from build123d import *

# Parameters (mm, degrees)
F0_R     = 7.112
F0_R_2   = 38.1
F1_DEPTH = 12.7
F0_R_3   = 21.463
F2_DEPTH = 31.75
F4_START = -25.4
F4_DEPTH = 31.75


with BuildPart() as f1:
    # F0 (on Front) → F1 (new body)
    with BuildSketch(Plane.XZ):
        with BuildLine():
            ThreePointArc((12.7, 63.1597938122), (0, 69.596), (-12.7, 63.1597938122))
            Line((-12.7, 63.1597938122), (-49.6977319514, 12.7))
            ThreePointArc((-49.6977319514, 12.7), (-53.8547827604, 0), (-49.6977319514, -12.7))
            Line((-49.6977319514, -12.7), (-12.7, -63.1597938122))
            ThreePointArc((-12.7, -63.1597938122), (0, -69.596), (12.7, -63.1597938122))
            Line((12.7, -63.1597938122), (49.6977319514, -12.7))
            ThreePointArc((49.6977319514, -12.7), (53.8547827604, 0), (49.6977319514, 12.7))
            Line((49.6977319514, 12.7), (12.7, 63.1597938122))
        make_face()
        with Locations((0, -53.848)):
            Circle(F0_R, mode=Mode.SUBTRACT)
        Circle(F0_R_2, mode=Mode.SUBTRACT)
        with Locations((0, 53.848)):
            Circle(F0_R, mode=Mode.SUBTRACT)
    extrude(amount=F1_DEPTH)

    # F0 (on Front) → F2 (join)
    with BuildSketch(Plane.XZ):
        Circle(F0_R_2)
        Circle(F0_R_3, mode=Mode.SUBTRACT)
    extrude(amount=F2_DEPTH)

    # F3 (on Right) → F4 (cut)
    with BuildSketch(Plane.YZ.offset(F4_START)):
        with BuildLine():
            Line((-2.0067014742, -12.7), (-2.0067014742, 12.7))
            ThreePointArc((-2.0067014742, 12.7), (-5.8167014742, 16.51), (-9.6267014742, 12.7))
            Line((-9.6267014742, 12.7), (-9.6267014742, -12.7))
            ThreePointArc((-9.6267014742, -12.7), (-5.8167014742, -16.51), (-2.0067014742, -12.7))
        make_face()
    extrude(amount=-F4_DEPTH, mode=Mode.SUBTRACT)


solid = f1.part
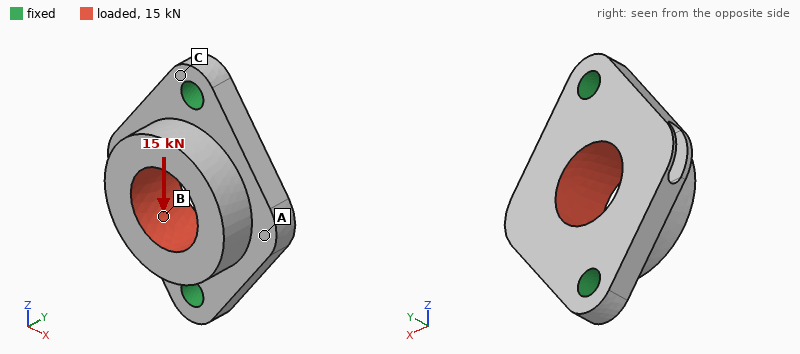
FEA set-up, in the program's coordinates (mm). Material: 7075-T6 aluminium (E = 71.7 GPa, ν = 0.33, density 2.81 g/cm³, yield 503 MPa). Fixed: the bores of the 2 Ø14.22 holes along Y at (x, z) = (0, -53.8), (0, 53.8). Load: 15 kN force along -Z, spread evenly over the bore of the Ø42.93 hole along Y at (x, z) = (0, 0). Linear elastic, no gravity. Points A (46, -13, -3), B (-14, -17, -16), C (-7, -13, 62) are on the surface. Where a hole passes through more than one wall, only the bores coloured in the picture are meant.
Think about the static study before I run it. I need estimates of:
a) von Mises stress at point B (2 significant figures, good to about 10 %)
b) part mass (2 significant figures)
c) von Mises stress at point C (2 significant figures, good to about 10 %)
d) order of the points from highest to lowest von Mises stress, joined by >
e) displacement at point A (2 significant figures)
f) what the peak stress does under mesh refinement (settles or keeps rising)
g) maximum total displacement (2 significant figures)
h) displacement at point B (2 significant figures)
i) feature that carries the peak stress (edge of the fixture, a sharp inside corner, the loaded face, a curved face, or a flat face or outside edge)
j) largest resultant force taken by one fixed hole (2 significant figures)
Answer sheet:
9.4 MPa
410 g
5.5 MPa
B > C > A
6.1 µm
keeps rising
11 µm
8.3 µm
edge of the fixture
7.7 kN
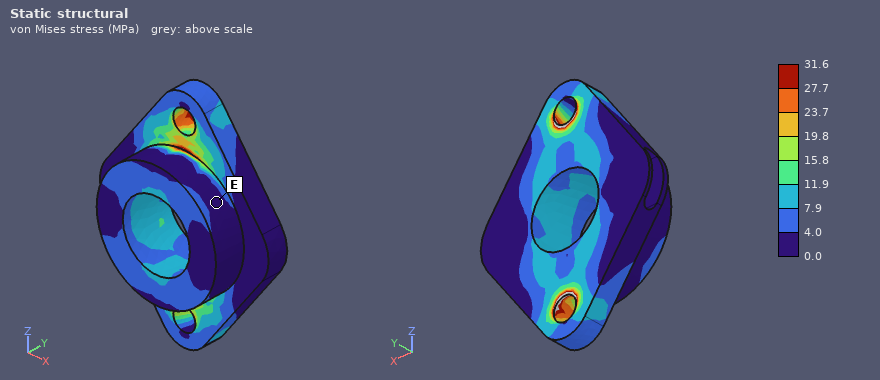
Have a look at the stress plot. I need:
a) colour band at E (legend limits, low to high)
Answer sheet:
0.0 to 4.0 MPa
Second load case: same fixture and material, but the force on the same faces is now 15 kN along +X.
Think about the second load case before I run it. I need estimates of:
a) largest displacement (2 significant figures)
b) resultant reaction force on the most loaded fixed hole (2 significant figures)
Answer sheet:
85 µm
7.5 kN
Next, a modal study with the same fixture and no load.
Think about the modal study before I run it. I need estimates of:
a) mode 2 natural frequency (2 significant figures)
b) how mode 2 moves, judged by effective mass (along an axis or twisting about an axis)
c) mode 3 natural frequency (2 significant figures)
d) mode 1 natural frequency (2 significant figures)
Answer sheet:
5000 Hz
along Y
8800 Hz
3000 Hz
